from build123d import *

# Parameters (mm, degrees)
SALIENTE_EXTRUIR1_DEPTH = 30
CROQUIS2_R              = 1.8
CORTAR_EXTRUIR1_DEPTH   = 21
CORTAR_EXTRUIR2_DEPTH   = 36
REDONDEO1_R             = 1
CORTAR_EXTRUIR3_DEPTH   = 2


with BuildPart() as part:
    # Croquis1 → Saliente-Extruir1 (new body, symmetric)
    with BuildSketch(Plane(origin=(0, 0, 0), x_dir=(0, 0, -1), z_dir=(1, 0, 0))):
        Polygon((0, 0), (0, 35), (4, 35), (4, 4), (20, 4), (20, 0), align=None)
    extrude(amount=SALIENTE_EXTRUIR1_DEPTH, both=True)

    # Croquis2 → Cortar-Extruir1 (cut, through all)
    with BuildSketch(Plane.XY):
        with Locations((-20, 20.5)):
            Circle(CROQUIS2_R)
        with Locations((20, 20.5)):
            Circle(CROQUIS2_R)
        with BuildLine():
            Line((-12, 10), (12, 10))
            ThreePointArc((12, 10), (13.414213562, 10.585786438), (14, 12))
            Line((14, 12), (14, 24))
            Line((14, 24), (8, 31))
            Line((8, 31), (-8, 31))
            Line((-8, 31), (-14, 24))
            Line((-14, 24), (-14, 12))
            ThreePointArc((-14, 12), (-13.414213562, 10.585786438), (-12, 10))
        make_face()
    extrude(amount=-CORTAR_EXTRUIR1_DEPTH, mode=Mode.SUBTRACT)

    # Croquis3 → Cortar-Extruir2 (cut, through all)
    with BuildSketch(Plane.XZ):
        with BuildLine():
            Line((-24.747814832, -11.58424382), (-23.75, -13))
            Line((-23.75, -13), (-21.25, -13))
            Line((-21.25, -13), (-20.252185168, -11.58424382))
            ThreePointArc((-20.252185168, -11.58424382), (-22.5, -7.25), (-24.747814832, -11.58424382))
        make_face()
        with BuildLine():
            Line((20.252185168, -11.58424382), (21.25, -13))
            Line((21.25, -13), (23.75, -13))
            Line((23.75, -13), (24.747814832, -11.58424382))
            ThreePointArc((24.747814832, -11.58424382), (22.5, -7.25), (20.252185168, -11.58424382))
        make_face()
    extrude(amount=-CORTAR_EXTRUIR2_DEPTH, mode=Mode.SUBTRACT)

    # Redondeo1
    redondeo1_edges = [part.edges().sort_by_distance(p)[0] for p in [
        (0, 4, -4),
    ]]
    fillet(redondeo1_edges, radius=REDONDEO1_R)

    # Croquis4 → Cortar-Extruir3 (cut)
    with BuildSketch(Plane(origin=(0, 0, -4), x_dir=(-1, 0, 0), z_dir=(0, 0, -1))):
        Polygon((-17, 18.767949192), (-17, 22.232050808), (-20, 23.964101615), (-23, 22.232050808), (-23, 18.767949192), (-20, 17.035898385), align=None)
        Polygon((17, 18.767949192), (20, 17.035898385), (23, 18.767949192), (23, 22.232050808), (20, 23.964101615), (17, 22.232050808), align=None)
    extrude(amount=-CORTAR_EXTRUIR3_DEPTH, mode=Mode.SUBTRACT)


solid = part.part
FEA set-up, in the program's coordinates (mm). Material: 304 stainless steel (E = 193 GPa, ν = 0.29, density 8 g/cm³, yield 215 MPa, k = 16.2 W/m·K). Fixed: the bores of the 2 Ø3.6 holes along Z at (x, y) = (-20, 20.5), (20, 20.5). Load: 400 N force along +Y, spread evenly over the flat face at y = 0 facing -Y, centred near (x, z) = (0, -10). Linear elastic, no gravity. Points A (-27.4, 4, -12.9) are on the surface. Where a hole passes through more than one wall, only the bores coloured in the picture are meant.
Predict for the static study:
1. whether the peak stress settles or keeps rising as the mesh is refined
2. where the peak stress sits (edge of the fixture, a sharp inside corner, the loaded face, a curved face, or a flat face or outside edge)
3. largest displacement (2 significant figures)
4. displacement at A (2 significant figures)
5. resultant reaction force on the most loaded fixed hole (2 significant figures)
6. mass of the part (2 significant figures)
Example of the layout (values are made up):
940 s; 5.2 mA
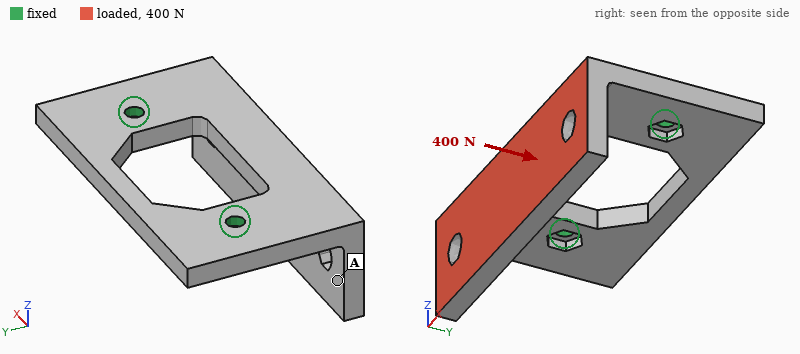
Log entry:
keeps rising; edge of the fixture; 59 µm; 36 µm; 210 N; 78 g
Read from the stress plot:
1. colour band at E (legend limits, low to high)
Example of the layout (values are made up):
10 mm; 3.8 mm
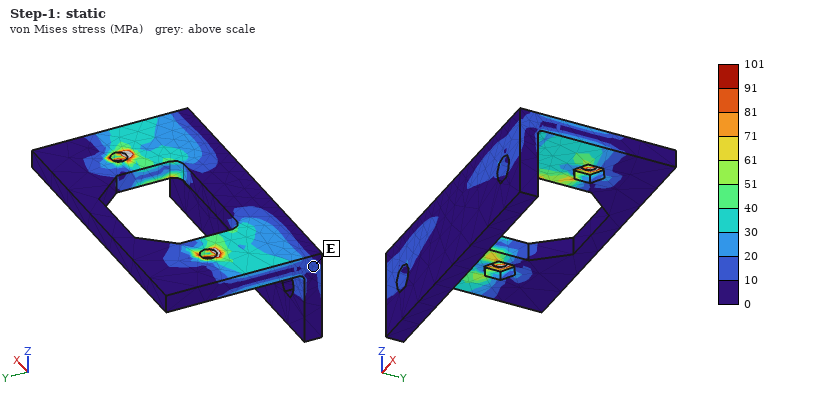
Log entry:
10 to 20 MPa
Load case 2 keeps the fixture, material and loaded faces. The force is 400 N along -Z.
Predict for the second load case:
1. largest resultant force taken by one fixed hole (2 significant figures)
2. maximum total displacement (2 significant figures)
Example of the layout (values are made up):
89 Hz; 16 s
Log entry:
200 N; 97 µm
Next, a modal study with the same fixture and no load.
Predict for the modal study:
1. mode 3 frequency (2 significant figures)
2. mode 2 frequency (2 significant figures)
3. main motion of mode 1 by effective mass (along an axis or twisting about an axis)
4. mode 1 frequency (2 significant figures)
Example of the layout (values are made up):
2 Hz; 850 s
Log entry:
6400 Hz; 3700 Hz; along Z; 1800 Hz
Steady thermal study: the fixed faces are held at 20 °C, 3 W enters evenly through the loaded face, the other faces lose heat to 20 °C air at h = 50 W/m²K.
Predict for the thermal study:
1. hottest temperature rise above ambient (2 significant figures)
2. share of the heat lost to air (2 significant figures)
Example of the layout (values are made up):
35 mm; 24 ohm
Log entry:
17 K; 66 %
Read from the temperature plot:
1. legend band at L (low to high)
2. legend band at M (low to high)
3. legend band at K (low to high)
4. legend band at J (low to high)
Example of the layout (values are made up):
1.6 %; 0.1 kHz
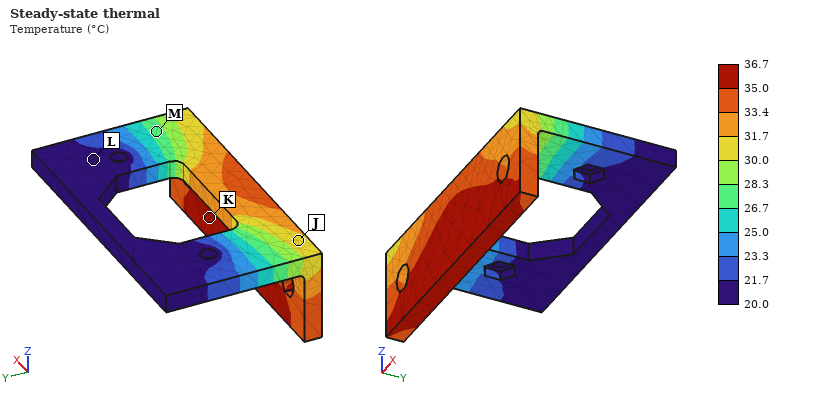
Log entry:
20.0 to 21.7 °C; 26.7 to 28.3 °C; 35.0 to 36.7 °C; 30.0 to 31.7 °C
